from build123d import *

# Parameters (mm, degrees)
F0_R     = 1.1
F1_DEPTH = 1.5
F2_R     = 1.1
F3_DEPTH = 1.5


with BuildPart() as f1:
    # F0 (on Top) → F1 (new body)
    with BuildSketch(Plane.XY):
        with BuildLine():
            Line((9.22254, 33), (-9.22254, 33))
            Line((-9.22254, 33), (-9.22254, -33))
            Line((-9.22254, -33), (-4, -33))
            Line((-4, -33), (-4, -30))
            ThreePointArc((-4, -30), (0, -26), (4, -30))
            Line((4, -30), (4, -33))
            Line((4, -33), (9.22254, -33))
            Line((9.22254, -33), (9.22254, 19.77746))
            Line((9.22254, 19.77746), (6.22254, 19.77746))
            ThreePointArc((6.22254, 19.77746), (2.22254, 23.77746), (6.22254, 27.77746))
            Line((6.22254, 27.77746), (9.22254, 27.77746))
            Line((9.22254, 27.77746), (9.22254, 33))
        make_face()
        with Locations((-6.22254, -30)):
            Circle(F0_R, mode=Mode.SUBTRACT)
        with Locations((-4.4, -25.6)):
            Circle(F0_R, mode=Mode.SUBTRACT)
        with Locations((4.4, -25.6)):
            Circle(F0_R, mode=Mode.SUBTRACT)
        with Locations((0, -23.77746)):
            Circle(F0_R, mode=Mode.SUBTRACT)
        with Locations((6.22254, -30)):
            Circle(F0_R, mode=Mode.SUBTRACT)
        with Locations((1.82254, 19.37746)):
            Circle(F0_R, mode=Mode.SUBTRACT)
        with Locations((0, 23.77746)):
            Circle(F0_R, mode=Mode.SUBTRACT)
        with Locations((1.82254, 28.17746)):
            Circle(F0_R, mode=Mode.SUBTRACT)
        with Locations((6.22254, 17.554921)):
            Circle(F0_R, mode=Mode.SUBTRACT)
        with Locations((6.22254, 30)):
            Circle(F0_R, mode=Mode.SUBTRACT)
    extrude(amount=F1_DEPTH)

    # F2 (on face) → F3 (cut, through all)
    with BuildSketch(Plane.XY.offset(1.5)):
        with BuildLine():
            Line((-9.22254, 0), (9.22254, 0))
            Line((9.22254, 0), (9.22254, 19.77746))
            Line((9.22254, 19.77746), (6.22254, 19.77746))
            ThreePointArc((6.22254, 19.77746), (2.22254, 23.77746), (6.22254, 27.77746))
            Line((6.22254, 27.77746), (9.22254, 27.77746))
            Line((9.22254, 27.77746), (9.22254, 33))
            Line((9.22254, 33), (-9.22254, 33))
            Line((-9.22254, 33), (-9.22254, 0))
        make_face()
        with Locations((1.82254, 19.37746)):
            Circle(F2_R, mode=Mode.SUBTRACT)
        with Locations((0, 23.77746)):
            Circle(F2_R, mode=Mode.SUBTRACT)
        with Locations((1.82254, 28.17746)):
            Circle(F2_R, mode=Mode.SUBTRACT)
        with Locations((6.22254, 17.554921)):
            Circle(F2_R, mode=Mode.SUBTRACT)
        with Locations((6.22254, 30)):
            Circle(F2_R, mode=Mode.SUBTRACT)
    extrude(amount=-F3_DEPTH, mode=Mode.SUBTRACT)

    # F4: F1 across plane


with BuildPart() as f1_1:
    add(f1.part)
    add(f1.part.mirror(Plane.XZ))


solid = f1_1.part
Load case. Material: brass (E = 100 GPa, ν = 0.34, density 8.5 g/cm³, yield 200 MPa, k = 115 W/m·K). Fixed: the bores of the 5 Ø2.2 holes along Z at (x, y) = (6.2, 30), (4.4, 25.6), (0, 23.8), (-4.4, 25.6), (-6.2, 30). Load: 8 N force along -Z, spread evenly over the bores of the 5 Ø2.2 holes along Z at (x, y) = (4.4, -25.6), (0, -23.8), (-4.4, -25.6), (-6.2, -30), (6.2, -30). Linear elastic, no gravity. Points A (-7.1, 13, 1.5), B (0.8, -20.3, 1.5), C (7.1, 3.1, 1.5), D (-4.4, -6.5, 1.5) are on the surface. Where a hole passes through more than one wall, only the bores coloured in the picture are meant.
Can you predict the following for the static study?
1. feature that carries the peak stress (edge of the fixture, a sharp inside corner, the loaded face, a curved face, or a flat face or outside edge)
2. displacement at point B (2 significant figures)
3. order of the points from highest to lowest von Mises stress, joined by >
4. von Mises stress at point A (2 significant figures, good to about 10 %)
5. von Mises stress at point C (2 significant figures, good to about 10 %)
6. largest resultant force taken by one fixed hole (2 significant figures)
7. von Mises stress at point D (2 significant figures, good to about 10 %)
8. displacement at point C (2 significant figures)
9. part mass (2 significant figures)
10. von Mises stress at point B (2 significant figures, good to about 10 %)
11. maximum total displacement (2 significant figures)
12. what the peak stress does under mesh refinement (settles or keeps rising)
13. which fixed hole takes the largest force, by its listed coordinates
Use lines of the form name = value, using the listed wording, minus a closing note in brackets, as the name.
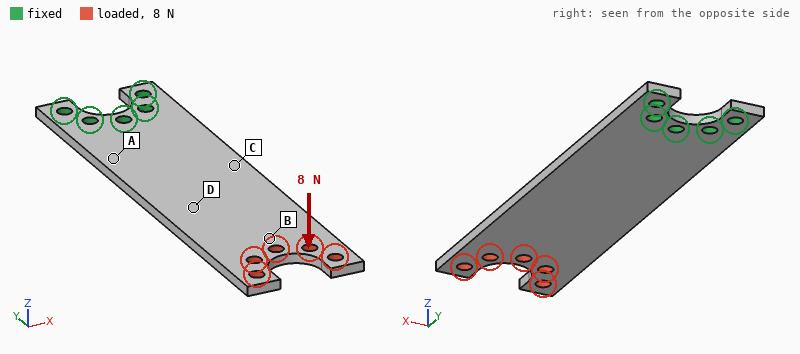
feature that carries the peak stress = edge of the fixture
displacement at point B = 0.53 mm
order of the points from highest to lowest von Mises stress, joined by > = A > C > D > B
von Mises stress at point A = 46 MPa
von Mises stress at point C = 35 MPa
largest resultant force taken by one fixed hole = 45 N
von Mises stress at point D = 24 MPa
displacement at point C = 0.14 mm
part mass = 14 g
von Mises stress at point B = 8.5 MPa
maximum total displacement = 0.77 mm
what the peak stress does under mesh refinement = keeps rising
which fixed hole takes the largest force, by its listed coordinates = (0, 23.8)
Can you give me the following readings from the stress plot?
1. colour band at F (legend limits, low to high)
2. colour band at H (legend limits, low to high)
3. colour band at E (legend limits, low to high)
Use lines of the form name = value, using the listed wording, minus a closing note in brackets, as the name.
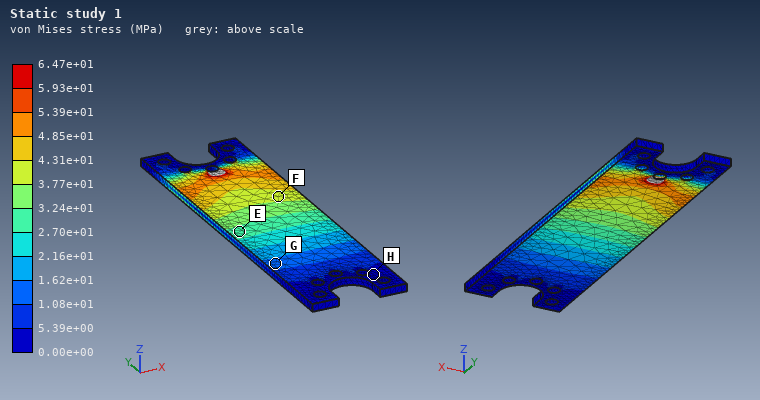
colour band at F = 3.77e+01 to 4.31e+01 MPa
colour band at H = 0.00e+00 to 5.39e+00 MPa
colour band at E = 2.70e+01 to 3.24e+01 MPa
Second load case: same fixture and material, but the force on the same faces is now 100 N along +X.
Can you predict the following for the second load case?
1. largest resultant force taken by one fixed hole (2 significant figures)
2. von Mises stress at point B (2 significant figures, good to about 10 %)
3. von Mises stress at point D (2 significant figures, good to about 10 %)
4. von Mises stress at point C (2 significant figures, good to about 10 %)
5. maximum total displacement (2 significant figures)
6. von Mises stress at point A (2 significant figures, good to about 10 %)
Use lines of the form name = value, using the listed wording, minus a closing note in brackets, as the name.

largest resultant force taken by one fixed hole = 290 N
von Mises stress at point B = 13 MPa
von Mises stress at point D = 14 MPa
von Mises stress at point C = 28 MPa
maximum total displacement = 88 µm
von Mises stress at point A = 36 MPa
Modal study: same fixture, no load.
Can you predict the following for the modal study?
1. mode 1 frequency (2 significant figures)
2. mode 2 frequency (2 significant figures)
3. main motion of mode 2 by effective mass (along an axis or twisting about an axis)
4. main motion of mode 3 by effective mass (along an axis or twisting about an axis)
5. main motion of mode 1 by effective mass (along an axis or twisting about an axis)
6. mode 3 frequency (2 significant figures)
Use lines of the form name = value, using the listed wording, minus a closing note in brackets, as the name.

mode 1 frequency = 300 Hz
mode 2 frequency = 1600 Hz
main motion of mode 2 by effective mass = twisting about Y
main motion of mode 3 by effective mass = along Z
main motion of mode 1 by effective mass = along Z
mode 3 frequency = 1800 Hz
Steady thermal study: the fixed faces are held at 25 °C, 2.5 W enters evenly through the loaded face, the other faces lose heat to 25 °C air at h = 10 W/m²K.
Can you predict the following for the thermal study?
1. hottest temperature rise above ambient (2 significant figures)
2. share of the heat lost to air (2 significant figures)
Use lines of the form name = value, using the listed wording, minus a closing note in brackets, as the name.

hottest temperature rise above ambient = 38 K
share of the heat lost to air = 17 %
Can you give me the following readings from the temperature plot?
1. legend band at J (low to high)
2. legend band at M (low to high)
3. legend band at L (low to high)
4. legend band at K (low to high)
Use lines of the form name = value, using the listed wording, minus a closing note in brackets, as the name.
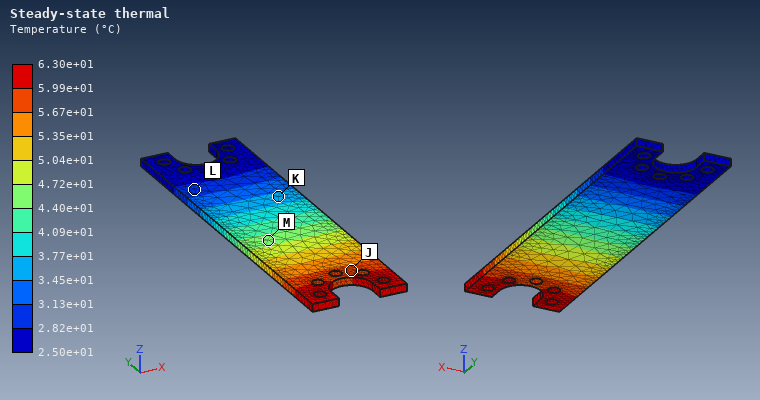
legend band at J = 5.67e+01 to 5.99e+01 °C
legend band at M = 4.40e+01 to 4.72e+01 °C
legend band at L = 2.82e+01 to 3.13e+01 °C
legend band at K = 3.45e+01 to 3.77e+01 °C
